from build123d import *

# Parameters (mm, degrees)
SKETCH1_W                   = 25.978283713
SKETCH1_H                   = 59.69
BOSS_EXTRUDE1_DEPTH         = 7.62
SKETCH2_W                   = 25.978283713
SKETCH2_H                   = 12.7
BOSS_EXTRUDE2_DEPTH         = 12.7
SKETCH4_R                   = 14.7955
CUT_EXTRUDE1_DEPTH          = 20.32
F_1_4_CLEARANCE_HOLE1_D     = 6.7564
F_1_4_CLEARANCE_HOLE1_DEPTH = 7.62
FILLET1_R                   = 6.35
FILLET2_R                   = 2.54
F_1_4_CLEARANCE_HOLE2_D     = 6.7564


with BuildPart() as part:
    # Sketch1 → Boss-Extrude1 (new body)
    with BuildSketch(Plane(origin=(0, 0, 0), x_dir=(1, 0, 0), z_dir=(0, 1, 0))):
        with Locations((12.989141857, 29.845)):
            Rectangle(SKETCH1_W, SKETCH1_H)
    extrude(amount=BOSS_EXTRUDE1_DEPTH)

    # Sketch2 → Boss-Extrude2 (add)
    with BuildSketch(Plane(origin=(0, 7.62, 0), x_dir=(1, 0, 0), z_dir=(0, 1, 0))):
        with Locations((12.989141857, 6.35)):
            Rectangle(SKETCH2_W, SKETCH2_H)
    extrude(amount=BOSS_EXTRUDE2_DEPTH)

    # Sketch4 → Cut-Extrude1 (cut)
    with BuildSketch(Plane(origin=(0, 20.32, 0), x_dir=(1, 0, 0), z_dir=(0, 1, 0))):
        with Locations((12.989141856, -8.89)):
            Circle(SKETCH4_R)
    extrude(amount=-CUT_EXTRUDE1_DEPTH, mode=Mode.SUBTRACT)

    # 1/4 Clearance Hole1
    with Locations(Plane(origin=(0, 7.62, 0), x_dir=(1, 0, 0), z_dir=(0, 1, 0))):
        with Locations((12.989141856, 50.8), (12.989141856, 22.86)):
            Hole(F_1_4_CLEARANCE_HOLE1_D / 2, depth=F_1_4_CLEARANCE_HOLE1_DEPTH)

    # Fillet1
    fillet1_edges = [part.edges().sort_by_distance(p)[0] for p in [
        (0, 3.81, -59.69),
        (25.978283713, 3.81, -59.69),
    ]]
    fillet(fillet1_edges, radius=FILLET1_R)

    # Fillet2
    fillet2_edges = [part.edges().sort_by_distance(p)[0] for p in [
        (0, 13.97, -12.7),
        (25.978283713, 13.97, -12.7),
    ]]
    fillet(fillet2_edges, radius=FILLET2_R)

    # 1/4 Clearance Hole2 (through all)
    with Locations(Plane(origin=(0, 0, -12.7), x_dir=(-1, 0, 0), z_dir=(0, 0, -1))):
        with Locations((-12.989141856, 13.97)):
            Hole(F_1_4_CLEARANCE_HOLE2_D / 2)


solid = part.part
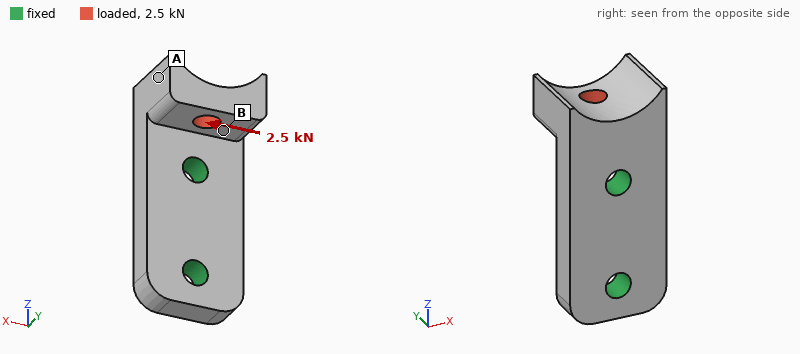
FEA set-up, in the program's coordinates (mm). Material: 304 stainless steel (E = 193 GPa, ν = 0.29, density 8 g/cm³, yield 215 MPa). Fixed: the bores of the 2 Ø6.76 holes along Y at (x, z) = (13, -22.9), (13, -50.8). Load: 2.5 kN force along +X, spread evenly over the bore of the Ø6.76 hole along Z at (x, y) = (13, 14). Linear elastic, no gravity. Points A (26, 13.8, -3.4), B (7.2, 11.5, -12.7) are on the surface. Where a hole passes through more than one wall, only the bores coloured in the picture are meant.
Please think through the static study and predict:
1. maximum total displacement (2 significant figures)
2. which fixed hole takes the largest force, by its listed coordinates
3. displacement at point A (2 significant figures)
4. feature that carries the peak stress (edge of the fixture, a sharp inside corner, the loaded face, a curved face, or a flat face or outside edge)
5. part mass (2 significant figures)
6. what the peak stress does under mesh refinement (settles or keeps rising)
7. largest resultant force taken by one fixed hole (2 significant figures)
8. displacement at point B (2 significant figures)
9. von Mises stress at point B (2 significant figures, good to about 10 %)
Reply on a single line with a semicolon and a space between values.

29 µm; (13, -22.9); 23 µm; edge of the fixture; 100 g; keeps rising; 3.2 kN; 14 µm; 45 MPa
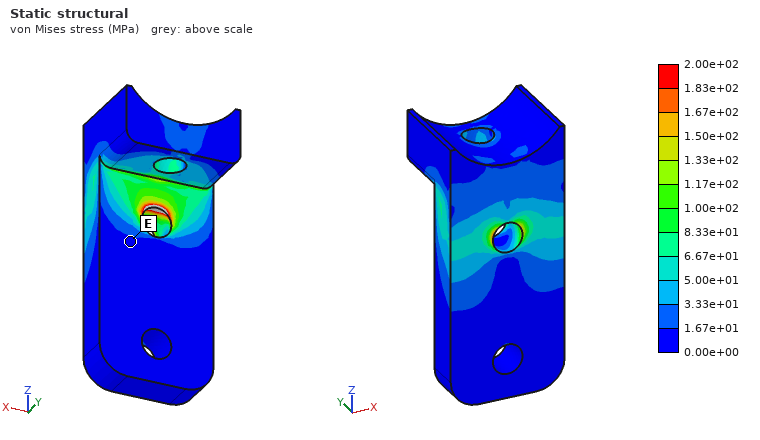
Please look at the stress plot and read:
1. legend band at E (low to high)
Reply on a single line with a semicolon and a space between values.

0.00e+00 to 1.67e+01 MPa
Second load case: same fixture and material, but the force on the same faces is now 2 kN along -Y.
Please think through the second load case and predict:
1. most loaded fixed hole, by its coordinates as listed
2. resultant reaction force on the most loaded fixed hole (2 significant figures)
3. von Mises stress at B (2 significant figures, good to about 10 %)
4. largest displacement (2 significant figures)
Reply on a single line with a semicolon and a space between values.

(13, -22.9); 2.2 kN; 20 MPa; 24 µm
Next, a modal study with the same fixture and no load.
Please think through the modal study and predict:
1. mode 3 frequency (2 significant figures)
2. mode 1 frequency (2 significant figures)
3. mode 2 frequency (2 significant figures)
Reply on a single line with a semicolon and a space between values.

15 kHz; 7800 Hz; 9900 Hz
